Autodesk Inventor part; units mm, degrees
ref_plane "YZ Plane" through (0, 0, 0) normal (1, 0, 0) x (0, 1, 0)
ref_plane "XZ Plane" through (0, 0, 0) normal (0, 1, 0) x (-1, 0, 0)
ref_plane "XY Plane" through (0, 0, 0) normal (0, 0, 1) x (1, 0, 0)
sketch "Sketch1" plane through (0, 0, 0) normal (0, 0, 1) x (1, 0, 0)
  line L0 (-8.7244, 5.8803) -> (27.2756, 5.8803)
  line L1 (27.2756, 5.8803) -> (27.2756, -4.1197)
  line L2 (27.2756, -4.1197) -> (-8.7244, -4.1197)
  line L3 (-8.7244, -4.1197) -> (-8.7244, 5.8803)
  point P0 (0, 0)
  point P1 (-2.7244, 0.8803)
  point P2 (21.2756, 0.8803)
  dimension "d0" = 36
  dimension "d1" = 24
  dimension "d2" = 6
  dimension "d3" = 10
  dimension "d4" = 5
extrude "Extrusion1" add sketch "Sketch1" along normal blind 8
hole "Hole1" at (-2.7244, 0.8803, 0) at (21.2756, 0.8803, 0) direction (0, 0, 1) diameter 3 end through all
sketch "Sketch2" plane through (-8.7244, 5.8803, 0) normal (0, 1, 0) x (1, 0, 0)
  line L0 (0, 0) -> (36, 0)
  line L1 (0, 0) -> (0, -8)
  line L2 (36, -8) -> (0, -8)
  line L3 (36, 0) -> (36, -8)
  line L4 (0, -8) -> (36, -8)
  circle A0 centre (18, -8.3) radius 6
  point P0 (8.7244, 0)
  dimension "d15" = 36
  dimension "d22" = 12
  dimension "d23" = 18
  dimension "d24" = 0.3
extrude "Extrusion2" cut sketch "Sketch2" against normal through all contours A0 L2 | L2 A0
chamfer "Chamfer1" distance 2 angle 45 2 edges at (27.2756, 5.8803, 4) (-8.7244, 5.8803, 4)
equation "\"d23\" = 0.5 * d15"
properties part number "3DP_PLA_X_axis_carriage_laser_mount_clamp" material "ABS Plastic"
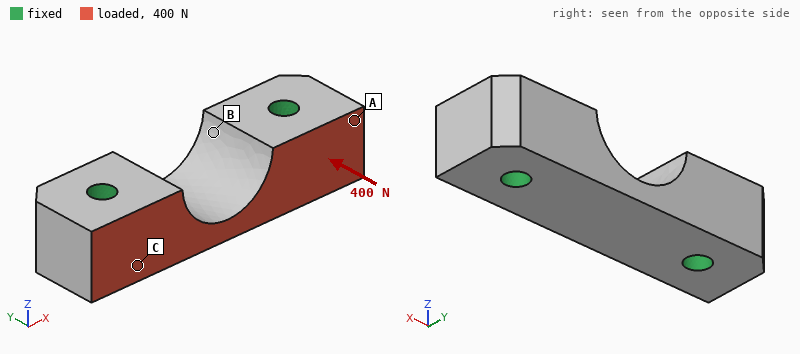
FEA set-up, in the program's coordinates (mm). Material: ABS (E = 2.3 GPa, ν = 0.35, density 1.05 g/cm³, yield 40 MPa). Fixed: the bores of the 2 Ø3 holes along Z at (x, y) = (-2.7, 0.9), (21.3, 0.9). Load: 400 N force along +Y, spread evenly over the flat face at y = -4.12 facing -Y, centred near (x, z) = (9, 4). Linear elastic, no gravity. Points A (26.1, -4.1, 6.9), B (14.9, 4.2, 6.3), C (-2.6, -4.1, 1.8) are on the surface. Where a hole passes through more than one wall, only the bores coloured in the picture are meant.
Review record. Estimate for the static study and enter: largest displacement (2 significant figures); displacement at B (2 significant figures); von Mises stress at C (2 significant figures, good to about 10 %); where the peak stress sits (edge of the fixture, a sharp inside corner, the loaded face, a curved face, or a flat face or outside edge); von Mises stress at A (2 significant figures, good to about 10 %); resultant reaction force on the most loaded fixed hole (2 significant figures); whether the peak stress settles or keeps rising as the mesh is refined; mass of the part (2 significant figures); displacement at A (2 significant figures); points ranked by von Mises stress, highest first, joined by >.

29 µm
12 µm
3.9 MPa
edge of the fixture
1.7 MPa
200 N
keeps rising
2.3 g
4.6 µm
C > A > B
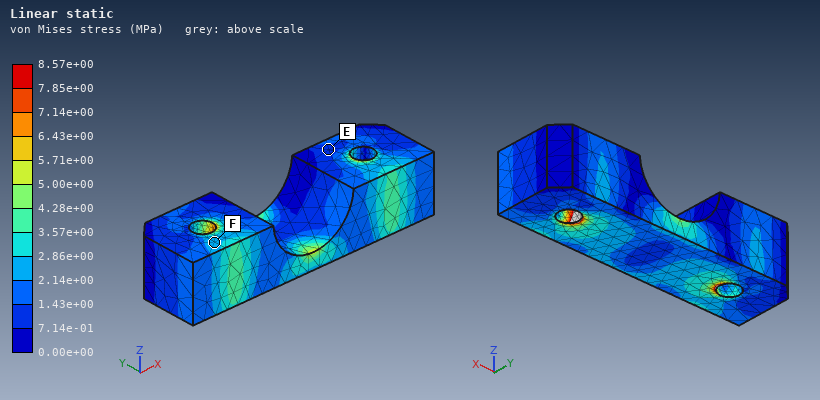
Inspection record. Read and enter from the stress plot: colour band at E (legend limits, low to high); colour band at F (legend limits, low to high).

7.14e-01 to 1.43e+00 MPa
2.14e+00 to 2.86e+00 MPa
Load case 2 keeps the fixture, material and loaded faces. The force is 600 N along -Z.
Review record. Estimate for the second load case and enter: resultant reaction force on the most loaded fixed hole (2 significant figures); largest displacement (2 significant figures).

300 N
0.10 mm
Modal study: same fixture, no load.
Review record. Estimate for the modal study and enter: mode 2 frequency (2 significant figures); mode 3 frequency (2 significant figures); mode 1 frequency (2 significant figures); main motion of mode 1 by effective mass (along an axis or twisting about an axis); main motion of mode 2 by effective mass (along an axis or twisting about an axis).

17 kHz
21 kHz
13 kHz
along Y
along Z
